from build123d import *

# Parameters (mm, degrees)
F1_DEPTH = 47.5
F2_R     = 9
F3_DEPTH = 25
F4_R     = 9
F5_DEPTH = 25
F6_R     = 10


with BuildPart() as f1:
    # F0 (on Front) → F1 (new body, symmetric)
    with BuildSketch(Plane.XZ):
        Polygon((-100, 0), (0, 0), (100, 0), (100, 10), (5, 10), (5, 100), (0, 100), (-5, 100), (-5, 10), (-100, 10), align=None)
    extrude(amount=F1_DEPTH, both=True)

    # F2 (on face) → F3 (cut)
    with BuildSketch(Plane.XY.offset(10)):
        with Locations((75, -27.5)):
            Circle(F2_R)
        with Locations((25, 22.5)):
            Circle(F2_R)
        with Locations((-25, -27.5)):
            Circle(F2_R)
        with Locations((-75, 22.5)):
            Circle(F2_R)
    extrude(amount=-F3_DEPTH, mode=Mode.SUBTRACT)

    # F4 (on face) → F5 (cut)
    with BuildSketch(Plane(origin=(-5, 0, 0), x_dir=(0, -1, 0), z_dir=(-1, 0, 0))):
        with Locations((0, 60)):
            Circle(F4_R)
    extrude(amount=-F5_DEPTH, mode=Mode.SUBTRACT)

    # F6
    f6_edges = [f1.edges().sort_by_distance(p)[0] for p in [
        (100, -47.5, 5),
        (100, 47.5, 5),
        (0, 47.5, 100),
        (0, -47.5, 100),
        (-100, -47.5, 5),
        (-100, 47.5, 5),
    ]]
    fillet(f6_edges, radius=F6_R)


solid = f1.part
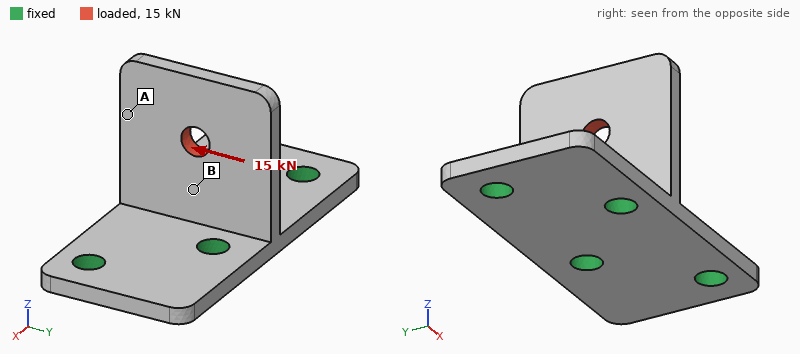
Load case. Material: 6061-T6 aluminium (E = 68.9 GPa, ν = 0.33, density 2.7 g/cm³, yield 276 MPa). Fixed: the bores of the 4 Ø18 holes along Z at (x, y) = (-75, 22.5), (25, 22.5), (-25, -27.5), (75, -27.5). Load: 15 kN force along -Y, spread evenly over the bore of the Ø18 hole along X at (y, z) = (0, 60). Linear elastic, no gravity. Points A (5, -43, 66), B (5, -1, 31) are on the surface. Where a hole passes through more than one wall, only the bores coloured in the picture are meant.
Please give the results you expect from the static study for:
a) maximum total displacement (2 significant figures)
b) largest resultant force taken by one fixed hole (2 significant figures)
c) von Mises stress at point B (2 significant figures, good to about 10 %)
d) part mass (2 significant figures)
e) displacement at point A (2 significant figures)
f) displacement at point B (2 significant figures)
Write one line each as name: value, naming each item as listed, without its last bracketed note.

maximum total displacement: 0.44 mm
largest resultant force taken by one fixed hole: 12 kN
von Mises stress at point B: 46 MPa
part mass: 710 g
displacement at point A: 0.31 mm
displacement at point B: 0.11 mm
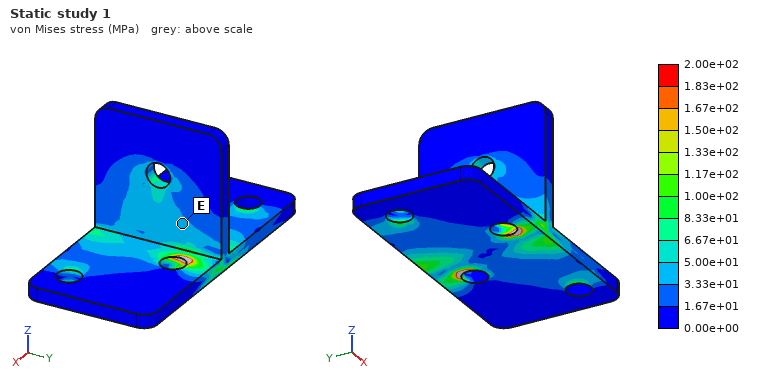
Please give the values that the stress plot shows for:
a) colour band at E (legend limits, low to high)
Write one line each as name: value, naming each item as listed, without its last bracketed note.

colour band at E: 3.33e+01 to 5.00e+01 MPa
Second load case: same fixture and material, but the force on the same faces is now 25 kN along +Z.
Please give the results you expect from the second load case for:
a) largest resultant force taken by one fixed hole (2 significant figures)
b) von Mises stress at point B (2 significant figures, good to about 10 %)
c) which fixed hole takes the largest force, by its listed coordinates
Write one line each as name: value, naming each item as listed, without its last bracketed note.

largest resultant force taken by one fixed hole: 13 kN
von Mises stress at point B: 39 MPa
which fixed hole takes the largest force, by its listed coordinates: (25, 22.5)
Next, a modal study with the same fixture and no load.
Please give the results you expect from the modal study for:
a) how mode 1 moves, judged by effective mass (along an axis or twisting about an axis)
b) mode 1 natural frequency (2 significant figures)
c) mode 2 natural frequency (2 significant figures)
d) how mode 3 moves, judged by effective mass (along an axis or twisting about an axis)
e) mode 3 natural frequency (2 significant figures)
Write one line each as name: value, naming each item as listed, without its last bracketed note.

how mode 1 moves, judged by effective mass: along X
mode 1 natural frequency: 880 Hz
mode 2 natural frequency: 2100 Hz
how mode 3 moves, judged by effective mass: along Y
mode 3 natural frequency: 2600 Hz
